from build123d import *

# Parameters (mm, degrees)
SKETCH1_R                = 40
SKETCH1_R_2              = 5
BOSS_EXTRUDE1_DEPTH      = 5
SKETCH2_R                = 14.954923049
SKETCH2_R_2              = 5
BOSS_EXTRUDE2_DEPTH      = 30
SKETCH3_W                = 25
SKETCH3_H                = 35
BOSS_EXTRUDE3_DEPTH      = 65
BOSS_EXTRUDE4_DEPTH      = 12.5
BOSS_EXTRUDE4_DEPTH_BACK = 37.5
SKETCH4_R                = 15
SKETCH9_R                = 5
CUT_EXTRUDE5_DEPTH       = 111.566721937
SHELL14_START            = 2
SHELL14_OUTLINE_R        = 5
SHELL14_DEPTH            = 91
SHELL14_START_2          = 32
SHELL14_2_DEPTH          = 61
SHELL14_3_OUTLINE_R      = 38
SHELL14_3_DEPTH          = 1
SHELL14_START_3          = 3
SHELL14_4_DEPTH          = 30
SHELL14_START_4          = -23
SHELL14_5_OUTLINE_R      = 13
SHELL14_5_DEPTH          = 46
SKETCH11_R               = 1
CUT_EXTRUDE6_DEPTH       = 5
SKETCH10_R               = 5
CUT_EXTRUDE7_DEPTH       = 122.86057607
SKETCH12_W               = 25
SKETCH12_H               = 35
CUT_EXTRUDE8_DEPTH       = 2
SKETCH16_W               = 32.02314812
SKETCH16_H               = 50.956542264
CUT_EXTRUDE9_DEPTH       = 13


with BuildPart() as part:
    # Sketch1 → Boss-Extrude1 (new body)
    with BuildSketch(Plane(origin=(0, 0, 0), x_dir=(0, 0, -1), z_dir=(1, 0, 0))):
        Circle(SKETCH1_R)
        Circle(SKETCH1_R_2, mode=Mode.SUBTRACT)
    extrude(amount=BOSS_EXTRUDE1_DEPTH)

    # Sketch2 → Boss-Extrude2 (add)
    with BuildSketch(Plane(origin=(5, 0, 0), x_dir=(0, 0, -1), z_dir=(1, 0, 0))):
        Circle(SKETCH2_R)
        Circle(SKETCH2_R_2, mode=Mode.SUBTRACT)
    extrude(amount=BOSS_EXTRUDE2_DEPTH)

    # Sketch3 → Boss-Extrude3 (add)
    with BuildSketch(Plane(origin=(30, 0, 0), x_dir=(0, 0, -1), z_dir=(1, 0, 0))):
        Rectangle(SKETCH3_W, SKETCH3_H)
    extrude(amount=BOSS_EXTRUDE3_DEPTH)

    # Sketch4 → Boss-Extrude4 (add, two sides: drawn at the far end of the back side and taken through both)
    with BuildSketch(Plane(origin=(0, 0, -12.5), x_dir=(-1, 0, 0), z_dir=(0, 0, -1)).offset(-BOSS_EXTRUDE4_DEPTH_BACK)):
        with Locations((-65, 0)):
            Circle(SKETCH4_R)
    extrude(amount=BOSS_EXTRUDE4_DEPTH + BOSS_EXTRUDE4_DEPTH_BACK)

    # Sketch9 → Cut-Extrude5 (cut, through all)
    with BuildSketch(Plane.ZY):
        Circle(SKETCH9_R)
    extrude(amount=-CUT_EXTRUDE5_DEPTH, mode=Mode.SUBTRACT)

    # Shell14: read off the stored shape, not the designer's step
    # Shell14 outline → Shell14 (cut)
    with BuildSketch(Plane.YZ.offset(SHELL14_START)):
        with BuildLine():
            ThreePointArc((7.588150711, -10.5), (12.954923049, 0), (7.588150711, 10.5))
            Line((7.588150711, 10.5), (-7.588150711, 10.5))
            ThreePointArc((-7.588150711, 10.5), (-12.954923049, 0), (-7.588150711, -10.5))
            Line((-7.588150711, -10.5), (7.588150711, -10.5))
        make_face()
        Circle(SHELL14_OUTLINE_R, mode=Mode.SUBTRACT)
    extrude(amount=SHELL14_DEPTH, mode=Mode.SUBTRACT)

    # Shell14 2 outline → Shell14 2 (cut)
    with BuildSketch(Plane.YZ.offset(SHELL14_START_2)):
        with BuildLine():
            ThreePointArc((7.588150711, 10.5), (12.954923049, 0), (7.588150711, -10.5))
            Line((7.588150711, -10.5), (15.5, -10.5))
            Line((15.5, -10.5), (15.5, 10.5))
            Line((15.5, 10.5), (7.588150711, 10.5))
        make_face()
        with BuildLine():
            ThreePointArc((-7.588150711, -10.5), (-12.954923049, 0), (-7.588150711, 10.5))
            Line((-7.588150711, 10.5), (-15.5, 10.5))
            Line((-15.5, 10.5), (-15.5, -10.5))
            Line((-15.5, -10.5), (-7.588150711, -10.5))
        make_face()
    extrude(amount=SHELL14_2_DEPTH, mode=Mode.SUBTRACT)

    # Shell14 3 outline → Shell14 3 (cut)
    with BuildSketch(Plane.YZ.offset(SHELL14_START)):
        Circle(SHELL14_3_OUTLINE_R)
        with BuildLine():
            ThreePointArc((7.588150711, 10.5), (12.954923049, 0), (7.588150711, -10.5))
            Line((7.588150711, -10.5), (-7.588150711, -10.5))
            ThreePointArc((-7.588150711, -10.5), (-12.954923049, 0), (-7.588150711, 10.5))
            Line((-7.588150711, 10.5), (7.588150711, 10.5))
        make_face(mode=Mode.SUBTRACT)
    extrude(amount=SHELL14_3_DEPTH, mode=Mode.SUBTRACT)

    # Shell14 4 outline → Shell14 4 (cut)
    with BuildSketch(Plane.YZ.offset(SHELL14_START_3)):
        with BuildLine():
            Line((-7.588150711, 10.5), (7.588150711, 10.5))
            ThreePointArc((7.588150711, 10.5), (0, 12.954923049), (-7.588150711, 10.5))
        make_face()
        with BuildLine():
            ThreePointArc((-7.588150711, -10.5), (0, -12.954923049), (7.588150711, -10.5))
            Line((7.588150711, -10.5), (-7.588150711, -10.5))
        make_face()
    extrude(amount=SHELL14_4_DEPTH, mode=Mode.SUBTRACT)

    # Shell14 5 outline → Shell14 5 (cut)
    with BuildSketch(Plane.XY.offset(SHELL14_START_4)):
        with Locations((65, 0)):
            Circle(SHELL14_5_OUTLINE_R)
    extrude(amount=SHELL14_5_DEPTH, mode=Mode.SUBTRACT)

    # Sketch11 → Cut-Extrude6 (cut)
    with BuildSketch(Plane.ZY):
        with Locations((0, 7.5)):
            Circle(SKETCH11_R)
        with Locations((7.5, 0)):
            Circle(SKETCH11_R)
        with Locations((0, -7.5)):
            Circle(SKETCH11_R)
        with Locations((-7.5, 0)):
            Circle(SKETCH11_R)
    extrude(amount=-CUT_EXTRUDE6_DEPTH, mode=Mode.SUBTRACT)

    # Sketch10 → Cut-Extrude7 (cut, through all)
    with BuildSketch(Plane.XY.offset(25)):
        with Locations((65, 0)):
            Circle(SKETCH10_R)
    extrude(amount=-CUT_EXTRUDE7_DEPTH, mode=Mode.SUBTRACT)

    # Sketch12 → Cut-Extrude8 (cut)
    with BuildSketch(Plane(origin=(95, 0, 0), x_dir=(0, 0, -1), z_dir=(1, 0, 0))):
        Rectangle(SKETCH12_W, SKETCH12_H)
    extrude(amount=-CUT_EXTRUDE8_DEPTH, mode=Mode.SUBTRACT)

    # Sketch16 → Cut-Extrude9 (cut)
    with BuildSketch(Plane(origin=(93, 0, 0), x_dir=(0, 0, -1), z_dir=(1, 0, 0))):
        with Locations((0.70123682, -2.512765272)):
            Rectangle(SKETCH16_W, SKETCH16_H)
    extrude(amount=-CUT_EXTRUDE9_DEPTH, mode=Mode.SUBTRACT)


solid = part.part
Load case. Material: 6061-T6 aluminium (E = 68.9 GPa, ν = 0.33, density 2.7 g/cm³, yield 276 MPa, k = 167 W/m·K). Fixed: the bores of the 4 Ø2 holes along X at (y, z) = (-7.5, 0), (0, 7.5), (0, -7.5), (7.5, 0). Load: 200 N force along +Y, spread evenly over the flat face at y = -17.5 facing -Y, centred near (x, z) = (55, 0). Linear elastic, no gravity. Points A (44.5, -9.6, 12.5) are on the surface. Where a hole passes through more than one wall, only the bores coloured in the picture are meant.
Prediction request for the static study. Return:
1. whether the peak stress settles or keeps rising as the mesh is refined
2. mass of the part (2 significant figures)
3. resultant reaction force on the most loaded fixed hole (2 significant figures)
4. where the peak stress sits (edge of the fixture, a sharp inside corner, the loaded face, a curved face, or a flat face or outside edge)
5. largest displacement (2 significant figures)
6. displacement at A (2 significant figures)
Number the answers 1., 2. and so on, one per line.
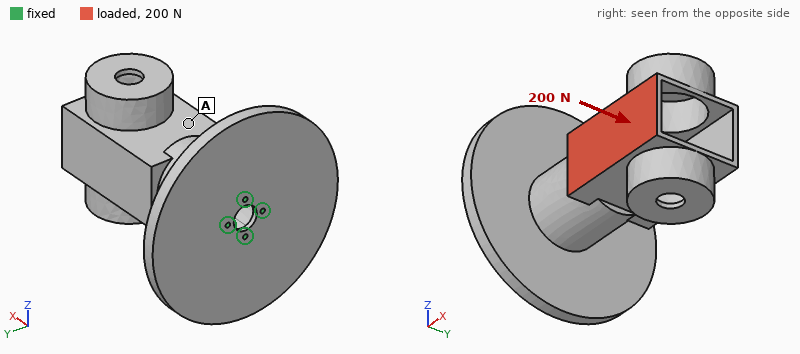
1. keeps rising
2. 110 g
3. 370 N
4. edge of the fixture
5. 1.5 mm
6. 0.84 mm
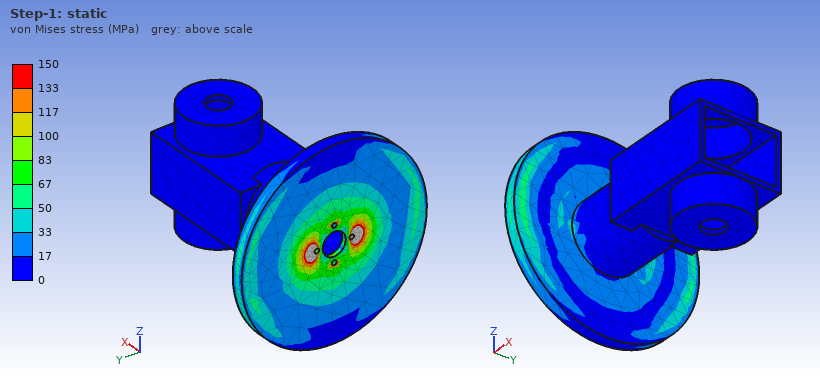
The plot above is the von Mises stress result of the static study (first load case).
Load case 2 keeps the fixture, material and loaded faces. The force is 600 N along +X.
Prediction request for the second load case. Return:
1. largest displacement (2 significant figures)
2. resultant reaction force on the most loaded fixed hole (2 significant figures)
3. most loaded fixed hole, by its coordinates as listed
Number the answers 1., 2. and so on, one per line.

1. 1.6 mm
2. 510 N
3. (-7.5, 0)
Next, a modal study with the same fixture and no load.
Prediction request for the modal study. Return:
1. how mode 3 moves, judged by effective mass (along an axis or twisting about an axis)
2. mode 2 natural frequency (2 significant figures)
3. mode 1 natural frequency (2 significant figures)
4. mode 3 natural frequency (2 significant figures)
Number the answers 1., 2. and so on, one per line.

1. along X
2. 290 Hz
3. 290 Hz
4. 770 Hz
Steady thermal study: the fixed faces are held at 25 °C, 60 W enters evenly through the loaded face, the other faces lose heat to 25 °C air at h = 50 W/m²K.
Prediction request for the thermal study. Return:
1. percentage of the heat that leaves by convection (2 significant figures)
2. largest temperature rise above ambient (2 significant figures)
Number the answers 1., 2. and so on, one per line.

1. 83 %
2. 74 K
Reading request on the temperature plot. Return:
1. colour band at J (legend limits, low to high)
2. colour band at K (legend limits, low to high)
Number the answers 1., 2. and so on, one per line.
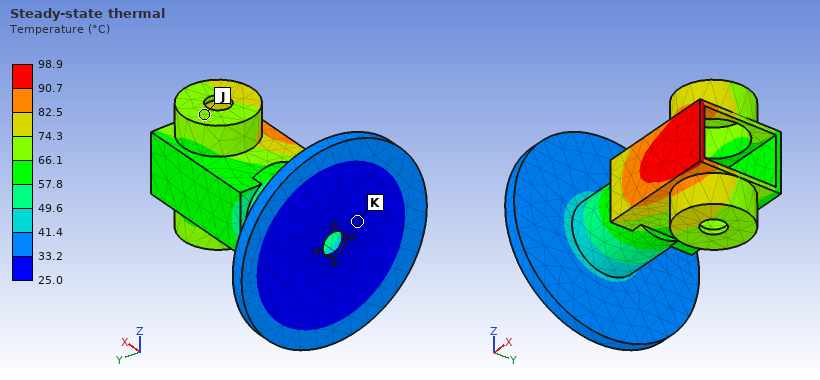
1. 66.1 to 74.3 °C
2. 25.0 to 33.2 °C
